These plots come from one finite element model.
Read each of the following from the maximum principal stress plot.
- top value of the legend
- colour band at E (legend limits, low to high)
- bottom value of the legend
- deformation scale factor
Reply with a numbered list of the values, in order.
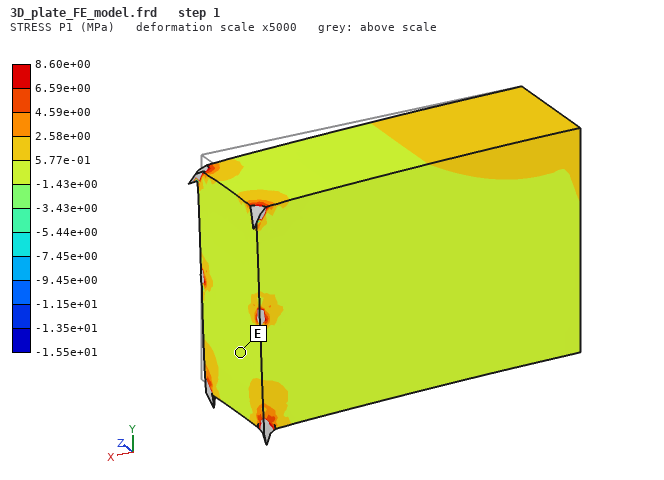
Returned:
1. 8.60e+00 MPa
2. -1.43e+00 to 5.77e-01 MPa
3. -1.55e+01 MPa
4. 5000
